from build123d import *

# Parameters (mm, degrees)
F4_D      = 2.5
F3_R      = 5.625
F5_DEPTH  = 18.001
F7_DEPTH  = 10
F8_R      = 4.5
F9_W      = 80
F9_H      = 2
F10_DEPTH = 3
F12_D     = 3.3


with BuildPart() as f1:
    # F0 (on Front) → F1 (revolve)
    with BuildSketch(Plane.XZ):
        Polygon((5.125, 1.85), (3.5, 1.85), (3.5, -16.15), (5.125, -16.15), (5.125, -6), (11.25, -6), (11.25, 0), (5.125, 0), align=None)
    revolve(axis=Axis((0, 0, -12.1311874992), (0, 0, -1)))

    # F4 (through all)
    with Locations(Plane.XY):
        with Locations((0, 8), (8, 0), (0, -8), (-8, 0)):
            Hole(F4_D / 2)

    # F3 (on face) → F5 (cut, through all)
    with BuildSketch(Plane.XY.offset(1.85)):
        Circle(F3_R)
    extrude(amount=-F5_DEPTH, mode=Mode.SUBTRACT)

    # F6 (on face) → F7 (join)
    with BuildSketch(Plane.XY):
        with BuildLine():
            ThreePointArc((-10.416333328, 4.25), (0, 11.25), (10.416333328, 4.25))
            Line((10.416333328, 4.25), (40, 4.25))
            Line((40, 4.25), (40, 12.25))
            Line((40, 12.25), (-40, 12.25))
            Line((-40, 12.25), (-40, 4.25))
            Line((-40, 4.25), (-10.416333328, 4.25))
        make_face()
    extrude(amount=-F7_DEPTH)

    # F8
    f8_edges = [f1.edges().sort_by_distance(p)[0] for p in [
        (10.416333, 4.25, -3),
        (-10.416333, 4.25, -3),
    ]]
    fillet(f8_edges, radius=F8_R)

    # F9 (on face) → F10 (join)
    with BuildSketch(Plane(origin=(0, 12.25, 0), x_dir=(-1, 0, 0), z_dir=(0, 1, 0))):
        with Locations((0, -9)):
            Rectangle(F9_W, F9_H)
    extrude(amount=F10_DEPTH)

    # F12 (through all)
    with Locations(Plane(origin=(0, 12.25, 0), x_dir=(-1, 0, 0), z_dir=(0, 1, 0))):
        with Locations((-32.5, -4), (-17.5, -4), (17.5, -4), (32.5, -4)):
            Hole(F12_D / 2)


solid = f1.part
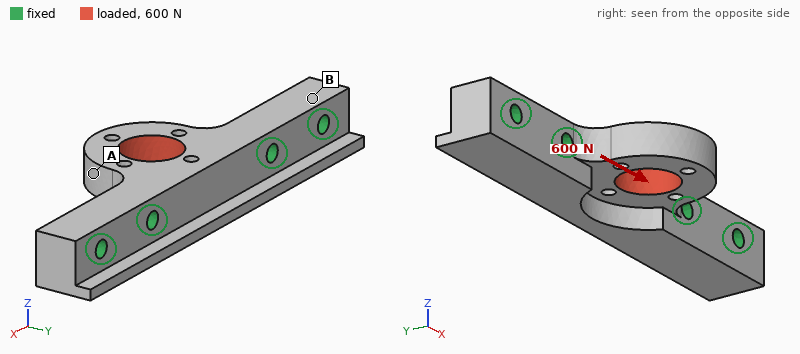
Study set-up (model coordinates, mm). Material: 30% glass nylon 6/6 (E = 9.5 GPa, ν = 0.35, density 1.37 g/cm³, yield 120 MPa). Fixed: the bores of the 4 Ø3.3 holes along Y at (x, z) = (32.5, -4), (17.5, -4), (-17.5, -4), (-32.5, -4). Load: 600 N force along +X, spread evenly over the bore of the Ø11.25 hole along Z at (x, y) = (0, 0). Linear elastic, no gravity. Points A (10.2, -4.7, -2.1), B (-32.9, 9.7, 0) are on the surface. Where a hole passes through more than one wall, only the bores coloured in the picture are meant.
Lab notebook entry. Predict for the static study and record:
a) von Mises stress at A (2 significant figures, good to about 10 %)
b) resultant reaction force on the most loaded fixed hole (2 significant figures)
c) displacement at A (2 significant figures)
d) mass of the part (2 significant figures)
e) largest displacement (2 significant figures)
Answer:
6.1 MPa
320 N
38 µm
10.0 g
45 µm
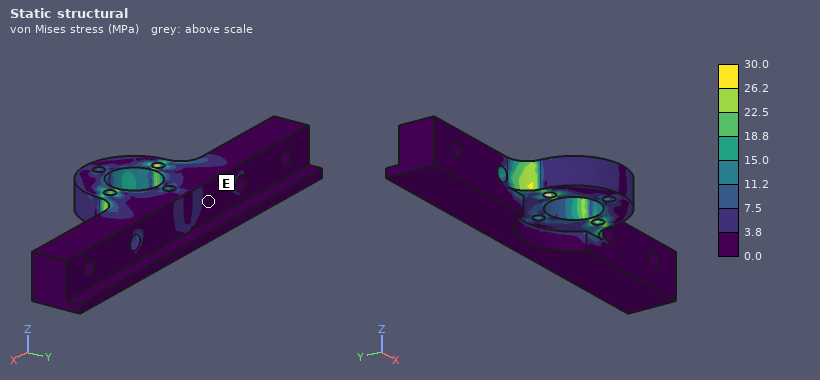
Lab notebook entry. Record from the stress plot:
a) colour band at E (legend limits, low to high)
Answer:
0.0 to 3.8 MPa
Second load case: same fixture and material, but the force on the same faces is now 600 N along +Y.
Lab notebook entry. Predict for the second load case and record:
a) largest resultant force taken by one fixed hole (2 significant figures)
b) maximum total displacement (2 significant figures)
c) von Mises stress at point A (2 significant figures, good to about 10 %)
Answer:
320 N
35 µm
3.9 MPa
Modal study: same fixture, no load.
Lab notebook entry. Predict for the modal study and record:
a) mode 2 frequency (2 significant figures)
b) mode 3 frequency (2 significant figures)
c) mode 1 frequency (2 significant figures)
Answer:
13 kHz
13 kHz
5600 Hz
